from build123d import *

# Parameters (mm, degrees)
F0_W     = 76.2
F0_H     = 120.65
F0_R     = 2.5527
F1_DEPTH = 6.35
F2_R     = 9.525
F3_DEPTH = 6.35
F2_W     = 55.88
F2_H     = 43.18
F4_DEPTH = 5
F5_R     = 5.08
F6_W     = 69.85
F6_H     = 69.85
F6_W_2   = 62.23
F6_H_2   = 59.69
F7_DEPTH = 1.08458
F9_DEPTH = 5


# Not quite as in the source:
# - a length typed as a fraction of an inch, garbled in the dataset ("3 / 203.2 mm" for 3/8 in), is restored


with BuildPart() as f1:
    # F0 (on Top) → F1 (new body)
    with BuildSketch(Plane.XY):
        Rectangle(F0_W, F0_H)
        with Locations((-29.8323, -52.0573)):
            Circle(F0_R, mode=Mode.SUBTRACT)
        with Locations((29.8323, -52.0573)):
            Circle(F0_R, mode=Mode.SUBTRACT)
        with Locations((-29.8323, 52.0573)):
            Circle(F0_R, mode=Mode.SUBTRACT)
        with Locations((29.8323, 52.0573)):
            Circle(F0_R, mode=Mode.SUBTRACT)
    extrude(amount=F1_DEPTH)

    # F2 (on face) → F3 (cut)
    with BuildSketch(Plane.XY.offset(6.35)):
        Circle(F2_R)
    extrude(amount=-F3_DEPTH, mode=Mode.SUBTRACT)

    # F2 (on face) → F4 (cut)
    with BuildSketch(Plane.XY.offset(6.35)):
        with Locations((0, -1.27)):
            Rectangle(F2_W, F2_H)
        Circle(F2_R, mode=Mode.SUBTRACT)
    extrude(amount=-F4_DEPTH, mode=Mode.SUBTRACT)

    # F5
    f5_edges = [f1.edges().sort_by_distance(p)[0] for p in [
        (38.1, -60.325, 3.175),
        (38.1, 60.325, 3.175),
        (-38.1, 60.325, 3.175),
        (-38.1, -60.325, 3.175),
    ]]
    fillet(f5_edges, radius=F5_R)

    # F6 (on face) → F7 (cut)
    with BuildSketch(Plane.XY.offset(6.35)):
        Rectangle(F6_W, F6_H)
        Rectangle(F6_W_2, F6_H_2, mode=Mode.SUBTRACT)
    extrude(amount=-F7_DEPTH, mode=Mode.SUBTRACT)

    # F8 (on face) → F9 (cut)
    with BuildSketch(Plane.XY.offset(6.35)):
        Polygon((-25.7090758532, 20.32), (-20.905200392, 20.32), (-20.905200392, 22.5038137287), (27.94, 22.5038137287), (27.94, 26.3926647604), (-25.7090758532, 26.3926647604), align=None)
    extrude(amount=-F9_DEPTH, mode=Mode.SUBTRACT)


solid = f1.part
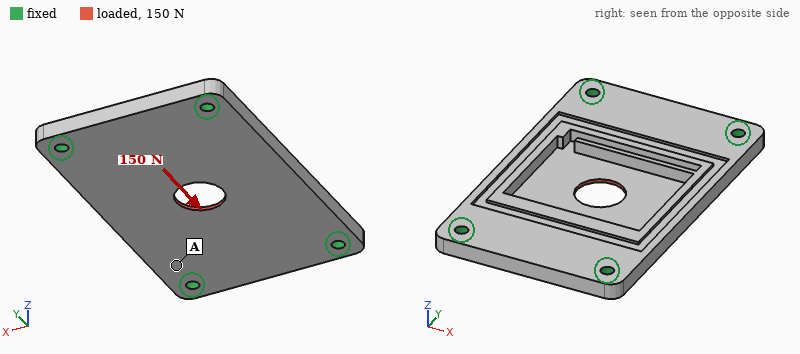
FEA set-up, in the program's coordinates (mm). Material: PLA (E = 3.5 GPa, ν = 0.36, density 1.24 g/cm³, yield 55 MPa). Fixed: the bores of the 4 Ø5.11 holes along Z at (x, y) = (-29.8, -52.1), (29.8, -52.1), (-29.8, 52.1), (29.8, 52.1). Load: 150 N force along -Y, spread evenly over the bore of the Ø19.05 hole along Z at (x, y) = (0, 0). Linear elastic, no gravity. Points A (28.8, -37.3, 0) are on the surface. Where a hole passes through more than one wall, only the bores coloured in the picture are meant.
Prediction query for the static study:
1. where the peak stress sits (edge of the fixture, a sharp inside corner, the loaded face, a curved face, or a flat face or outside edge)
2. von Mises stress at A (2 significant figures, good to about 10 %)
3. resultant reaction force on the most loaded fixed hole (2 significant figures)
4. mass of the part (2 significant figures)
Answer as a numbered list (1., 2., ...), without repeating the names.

1. the loaded face
2. 0.44 MPa
3. 40 N
4. 53 g
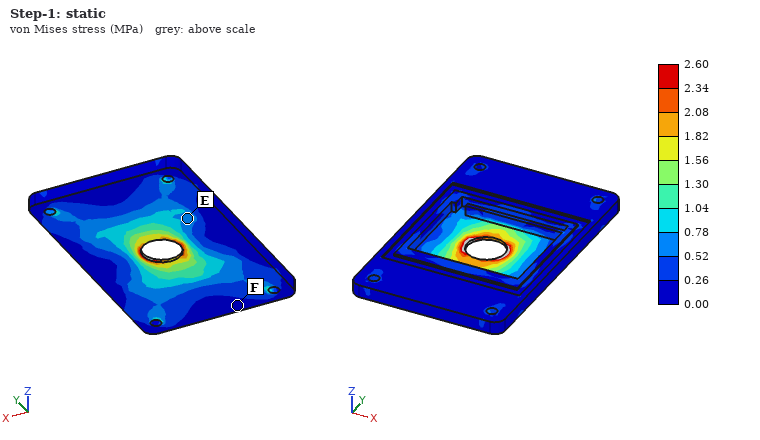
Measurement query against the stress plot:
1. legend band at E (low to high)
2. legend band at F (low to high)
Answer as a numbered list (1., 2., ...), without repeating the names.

1. 0.52 to 0.78 MPa
2. 0.00 to 0.26 MPa
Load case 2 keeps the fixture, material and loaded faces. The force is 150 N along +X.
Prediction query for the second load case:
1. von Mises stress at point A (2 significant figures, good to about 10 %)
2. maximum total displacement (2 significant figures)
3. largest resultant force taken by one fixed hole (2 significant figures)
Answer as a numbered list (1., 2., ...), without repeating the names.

1. 0.37 MPa
2. 22 µm
3. 51 N
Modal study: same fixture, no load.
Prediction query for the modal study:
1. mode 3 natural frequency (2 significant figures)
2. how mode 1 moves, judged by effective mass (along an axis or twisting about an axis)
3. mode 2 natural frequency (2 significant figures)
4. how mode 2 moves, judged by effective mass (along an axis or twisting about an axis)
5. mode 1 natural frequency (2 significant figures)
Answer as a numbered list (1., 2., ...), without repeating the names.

1. 1700 Hz
2. along Z
3. 1300 Hz
4. twisting about Y
5. 1000 Hz
